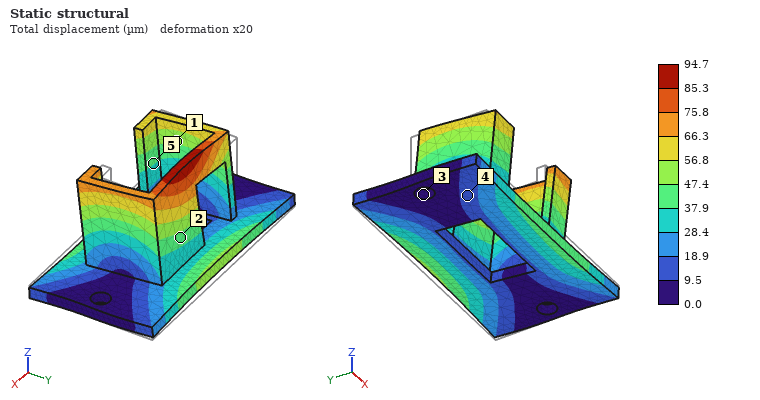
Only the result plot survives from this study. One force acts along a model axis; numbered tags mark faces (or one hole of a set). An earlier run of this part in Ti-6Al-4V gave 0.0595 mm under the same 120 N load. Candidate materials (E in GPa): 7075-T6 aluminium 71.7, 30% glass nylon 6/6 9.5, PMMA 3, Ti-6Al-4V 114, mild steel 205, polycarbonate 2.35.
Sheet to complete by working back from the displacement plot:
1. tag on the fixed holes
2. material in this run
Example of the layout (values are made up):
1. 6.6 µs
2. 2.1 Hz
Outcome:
1. 3
2. 7075-T6 aluminium
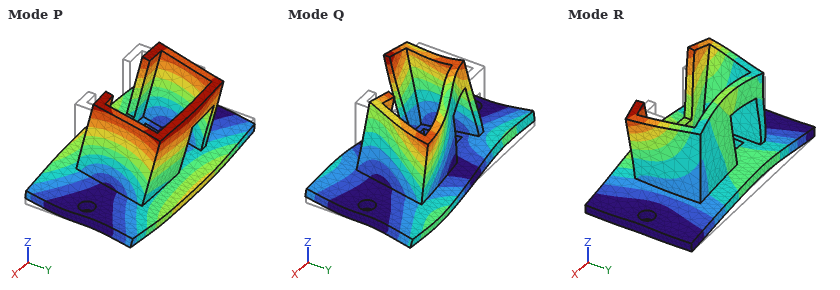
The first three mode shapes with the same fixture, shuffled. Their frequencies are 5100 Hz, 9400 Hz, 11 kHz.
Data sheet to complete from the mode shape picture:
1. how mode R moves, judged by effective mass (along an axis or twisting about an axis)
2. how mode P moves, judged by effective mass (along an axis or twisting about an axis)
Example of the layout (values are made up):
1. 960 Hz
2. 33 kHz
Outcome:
1. along Z
2. along Y
